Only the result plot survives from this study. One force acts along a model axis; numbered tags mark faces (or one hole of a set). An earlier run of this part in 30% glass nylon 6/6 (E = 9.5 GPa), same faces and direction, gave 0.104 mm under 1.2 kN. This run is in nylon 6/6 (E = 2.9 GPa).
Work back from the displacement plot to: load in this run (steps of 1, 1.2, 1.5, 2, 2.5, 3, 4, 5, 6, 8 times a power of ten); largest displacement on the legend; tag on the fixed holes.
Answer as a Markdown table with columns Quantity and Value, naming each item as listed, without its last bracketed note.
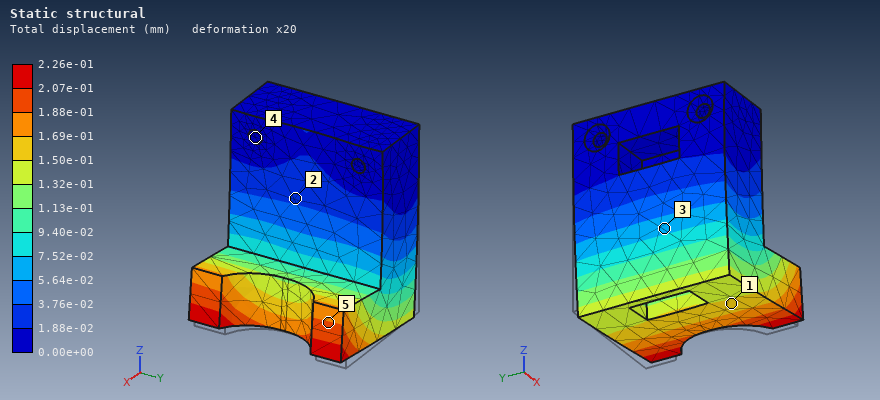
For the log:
| Quantity | Value |
|---|---|
| load in this run | 800 N |
| largest displacement on the legend | 2.26e-01 mm |
| tag on the fixed holes | 4 |
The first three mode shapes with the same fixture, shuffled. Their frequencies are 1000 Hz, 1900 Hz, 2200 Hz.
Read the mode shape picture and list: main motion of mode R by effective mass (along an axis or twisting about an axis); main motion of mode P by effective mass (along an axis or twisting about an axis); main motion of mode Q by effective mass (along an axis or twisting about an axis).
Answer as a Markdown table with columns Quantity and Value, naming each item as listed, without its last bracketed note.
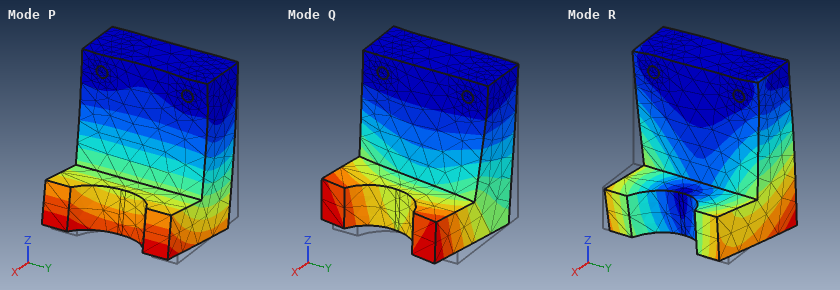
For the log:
| Quantity | Value |
|---|---|
| main motion of mode R by effective mass | along Y |
| main motion of mode P by effective mass | along X |
| main motion of mode Q by effective mass | along Y |
